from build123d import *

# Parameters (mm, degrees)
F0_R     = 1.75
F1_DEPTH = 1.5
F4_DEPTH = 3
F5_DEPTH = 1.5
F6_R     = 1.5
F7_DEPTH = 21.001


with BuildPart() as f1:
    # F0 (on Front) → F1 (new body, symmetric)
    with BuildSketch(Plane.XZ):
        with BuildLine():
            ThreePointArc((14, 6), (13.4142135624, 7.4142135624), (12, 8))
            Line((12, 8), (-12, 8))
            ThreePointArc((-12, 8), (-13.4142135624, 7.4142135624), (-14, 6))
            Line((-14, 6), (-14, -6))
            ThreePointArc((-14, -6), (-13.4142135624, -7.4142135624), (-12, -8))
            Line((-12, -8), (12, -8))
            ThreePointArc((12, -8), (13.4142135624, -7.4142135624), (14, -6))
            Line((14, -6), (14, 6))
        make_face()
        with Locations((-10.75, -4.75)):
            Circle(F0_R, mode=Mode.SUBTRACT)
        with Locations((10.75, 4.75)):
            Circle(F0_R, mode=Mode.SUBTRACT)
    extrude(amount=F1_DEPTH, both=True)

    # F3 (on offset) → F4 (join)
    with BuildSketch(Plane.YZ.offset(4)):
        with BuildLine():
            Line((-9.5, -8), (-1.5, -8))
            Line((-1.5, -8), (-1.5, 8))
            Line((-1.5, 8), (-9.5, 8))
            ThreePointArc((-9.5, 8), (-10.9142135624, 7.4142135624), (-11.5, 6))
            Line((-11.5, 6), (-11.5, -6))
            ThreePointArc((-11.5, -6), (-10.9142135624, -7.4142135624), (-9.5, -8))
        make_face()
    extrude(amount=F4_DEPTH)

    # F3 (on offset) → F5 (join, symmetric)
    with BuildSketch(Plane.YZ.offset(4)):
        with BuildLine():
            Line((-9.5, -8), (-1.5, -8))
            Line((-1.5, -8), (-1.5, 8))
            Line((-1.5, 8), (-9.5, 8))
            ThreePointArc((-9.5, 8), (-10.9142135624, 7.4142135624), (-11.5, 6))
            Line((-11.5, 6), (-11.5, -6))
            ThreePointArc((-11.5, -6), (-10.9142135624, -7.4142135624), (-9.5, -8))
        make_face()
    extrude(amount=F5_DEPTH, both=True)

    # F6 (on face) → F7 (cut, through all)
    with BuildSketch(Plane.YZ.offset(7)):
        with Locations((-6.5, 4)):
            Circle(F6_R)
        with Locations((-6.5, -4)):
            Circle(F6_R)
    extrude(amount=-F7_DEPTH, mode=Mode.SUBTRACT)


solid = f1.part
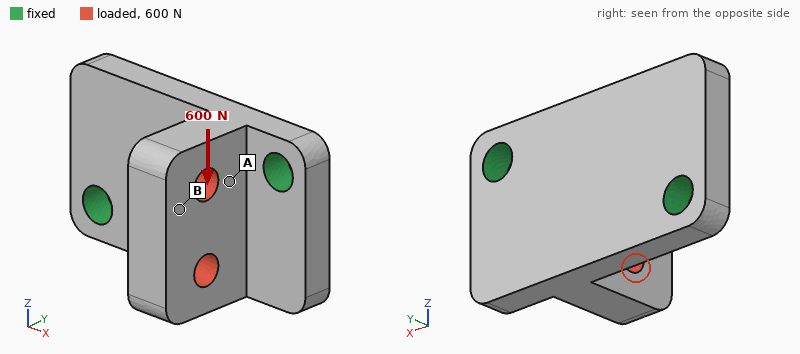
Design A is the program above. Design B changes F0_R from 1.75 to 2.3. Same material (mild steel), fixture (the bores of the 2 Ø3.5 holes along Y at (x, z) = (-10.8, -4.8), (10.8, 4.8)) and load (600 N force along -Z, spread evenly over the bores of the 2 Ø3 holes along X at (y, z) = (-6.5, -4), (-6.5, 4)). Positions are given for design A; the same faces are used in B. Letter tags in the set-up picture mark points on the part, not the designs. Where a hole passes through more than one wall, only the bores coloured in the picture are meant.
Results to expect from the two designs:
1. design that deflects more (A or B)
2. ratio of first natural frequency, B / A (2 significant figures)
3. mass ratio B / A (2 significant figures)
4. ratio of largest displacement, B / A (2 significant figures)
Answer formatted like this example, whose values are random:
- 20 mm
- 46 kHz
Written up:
- A
- 1.1
- 0.98
- 0.80
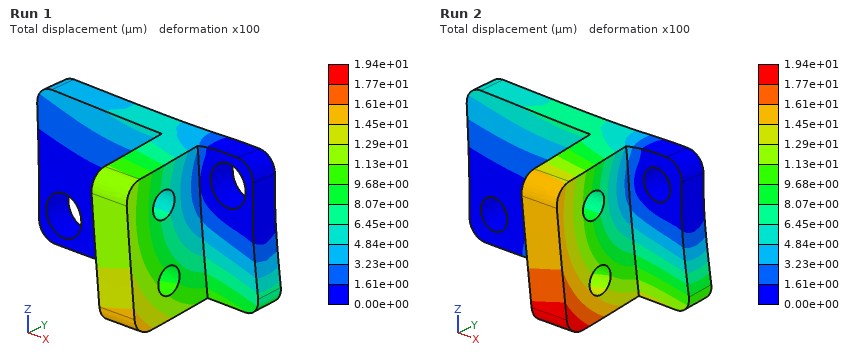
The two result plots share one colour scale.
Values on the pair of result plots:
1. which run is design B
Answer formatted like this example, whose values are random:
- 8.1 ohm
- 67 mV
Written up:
- Run 1
